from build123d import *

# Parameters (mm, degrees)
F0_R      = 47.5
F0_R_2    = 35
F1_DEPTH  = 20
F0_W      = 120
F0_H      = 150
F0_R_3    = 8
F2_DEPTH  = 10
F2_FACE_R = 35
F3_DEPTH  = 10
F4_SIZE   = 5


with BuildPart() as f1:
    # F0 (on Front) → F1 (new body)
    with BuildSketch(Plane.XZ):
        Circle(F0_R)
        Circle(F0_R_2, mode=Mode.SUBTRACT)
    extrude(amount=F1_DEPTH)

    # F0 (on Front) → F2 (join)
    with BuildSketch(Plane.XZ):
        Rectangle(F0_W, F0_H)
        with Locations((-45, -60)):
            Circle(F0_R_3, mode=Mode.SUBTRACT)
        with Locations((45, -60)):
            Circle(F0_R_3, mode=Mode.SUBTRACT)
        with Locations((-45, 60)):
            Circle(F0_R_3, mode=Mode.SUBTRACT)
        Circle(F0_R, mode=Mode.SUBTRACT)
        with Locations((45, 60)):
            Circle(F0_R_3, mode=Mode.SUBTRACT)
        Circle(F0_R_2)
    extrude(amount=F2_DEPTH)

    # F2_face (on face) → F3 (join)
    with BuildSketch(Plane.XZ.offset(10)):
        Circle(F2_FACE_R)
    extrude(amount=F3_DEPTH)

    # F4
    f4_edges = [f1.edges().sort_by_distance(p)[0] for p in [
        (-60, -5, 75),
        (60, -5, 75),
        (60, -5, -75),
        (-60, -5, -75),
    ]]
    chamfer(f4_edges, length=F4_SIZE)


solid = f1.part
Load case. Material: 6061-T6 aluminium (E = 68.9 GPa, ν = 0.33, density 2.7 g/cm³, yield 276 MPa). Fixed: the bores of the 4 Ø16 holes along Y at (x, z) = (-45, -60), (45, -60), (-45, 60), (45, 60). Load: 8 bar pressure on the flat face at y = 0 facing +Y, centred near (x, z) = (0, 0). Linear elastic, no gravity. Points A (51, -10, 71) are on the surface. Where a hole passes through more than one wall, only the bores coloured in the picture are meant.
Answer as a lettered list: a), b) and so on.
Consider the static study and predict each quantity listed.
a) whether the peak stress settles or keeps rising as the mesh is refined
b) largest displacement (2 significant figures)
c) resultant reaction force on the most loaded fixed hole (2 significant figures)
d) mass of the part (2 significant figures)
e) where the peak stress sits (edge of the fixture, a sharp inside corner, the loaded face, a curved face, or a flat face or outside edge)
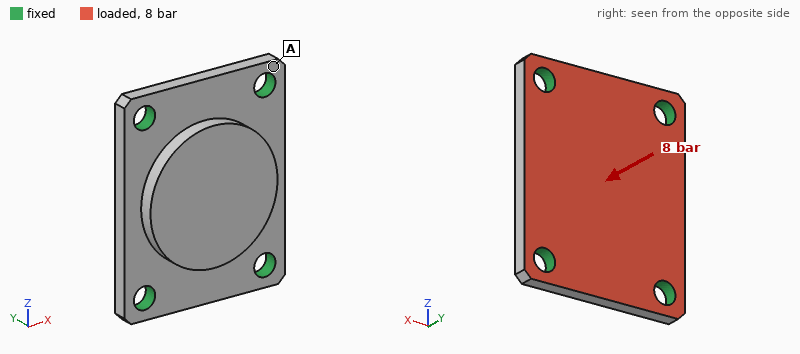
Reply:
a) keeps rising
b) 39 µm
c) 3.6 kN
d) 650 g
e) edge of the fixture
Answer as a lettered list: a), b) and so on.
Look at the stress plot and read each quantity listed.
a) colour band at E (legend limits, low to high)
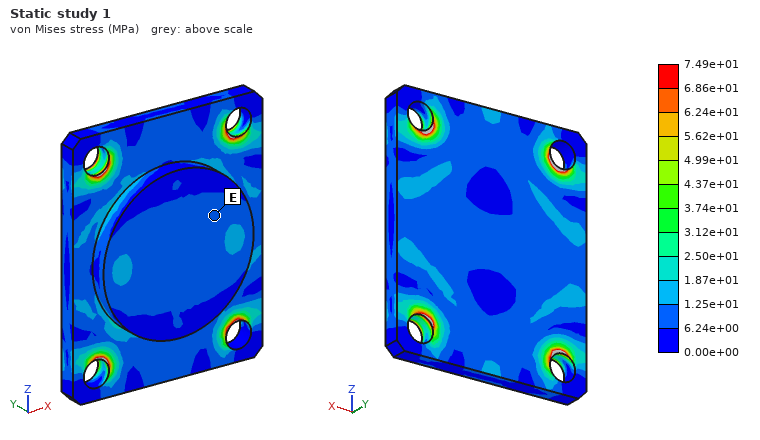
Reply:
a) 6.24e+00 to 1.25e+01 MPa
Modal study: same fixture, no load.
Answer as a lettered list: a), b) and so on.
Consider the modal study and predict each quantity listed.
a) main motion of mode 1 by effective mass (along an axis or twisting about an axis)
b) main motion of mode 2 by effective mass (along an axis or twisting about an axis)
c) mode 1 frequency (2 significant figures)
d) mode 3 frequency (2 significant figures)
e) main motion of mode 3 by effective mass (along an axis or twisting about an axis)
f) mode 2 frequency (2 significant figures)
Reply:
a) along Y
b) twisting about Z
c) 3900 Hz
d) 7400 Hz
e) twisting about X
f) 5200 Hz
